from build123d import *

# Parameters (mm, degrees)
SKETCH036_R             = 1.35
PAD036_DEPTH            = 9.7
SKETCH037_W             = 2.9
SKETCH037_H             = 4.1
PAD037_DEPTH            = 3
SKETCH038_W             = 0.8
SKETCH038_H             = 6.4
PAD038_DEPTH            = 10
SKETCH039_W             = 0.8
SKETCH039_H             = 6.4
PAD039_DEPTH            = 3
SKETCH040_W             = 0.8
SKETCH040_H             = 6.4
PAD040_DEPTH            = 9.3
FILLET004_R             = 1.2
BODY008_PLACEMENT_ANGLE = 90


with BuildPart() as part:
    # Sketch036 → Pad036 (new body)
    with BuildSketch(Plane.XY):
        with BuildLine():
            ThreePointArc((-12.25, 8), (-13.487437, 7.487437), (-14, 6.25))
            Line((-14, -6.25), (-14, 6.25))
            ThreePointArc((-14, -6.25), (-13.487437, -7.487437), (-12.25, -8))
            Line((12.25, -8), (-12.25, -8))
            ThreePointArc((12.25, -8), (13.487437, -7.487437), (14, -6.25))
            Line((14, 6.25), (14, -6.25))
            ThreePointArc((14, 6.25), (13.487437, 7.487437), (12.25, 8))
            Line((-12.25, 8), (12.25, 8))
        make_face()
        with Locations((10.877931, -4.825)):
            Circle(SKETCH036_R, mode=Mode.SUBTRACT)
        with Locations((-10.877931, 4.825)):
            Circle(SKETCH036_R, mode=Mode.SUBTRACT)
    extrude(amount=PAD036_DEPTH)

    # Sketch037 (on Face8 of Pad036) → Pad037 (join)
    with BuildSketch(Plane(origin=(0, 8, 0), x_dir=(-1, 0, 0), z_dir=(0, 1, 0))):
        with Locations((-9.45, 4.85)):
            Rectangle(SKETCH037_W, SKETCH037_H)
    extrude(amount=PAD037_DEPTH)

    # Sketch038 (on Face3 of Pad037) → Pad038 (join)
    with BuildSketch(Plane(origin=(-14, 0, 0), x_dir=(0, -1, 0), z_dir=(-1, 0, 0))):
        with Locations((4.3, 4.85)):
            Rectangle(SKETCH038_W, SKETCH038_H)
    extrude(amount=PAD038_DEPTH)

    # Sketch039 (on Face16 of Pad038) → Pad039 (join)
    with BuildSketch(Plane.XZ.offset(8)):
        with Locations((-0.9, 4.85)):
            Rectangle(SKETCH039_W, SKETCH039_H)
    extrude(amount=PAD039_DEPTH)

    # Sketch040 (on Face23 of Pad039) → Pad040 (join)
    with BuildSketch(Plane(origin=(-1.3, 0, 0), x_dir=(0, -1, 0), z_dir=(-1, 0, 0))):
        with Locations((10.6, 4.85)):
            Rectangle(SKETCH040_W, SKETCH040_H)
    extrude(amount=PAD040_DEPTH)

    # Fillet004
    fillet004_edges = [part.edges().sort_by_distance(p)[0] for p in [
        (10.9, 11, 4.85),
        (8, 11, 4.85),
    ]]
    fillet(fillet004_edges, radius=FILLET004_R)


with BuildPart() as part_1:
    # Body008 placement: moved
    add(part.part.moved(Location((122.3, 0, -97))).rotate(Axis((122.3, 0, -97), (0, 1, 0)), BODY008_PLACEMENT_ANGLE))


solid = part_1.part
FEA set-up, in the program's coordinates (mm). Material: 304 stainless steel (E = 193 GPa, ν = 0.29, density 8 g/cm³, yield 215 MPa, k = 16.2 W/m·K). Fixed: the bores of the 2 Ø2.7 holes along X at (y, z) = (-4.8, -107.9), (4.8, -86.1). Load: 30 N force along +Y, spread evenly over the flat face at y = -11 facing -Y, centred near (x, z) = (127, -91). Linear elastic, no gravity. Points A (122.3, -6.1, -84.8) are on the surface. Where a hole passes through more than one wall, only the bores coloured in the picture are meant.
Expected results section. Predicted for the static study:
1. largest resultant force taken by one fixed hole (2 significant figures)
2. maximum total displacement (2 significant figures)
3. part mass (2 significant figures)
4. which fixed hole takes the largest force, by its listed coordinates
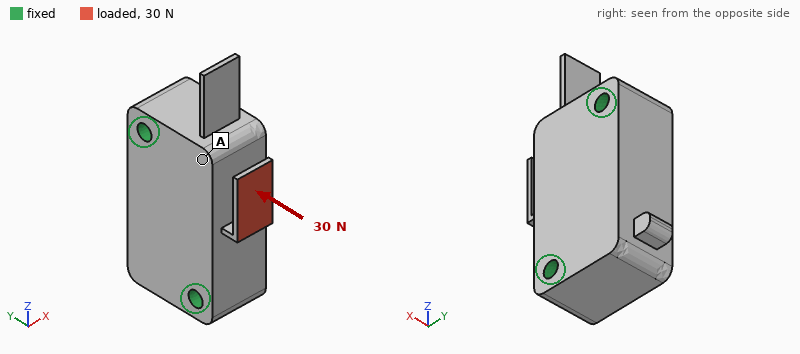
23 N
0.12 mm
35 g
(4.8, -86.1)
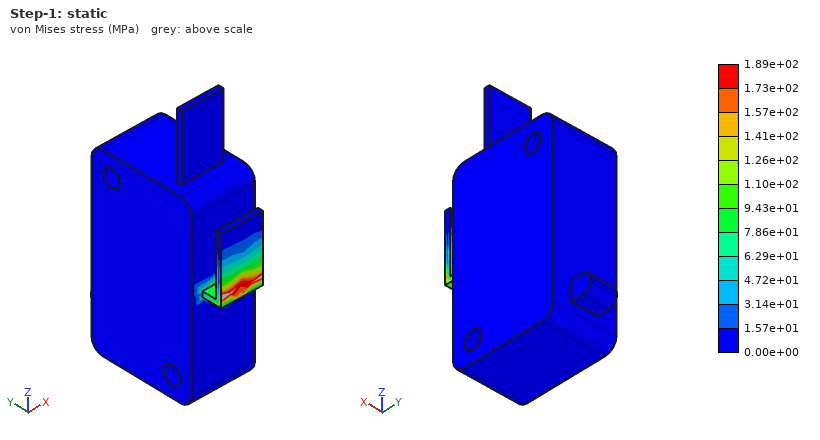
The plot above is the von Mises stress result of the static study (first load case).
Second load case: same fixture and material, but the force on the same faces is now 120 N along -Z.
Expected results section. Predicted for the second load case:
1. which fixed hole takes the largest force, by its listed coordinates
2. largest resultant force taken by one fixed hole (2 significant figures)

(-4.8, -107.9)
94 N
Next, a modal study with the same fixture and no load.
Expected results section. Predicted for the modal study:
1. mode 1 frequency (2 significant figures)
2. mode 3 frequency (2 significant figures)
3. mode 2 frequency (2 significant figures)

4900 Hz
12 kHz
6200 Hz
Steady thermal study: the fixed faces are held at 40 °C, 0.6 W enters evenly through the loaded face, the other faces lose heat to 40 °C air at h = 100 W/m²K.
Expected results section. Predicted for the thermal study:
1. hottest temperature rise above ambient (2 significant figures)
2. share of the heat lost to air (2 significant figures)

32 K
54 %
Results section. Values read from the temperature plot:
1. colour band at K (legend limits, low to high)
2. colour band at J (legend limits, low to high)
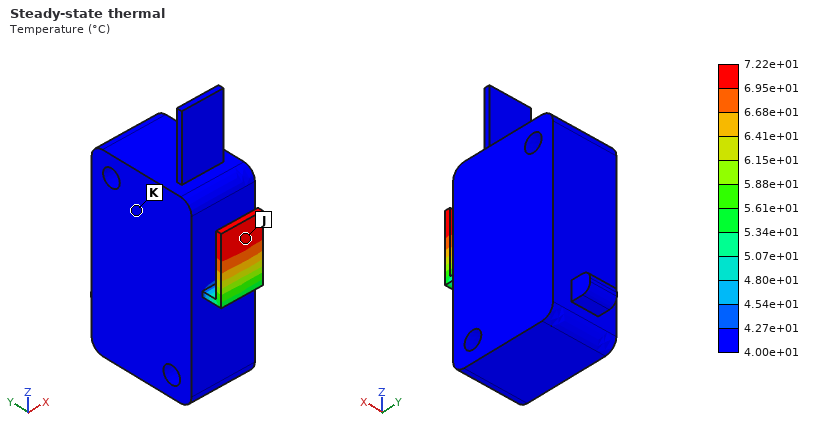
4.00e+01 to 4.27e+01 °C
6.95e+01 to 7.22e+01 °C
